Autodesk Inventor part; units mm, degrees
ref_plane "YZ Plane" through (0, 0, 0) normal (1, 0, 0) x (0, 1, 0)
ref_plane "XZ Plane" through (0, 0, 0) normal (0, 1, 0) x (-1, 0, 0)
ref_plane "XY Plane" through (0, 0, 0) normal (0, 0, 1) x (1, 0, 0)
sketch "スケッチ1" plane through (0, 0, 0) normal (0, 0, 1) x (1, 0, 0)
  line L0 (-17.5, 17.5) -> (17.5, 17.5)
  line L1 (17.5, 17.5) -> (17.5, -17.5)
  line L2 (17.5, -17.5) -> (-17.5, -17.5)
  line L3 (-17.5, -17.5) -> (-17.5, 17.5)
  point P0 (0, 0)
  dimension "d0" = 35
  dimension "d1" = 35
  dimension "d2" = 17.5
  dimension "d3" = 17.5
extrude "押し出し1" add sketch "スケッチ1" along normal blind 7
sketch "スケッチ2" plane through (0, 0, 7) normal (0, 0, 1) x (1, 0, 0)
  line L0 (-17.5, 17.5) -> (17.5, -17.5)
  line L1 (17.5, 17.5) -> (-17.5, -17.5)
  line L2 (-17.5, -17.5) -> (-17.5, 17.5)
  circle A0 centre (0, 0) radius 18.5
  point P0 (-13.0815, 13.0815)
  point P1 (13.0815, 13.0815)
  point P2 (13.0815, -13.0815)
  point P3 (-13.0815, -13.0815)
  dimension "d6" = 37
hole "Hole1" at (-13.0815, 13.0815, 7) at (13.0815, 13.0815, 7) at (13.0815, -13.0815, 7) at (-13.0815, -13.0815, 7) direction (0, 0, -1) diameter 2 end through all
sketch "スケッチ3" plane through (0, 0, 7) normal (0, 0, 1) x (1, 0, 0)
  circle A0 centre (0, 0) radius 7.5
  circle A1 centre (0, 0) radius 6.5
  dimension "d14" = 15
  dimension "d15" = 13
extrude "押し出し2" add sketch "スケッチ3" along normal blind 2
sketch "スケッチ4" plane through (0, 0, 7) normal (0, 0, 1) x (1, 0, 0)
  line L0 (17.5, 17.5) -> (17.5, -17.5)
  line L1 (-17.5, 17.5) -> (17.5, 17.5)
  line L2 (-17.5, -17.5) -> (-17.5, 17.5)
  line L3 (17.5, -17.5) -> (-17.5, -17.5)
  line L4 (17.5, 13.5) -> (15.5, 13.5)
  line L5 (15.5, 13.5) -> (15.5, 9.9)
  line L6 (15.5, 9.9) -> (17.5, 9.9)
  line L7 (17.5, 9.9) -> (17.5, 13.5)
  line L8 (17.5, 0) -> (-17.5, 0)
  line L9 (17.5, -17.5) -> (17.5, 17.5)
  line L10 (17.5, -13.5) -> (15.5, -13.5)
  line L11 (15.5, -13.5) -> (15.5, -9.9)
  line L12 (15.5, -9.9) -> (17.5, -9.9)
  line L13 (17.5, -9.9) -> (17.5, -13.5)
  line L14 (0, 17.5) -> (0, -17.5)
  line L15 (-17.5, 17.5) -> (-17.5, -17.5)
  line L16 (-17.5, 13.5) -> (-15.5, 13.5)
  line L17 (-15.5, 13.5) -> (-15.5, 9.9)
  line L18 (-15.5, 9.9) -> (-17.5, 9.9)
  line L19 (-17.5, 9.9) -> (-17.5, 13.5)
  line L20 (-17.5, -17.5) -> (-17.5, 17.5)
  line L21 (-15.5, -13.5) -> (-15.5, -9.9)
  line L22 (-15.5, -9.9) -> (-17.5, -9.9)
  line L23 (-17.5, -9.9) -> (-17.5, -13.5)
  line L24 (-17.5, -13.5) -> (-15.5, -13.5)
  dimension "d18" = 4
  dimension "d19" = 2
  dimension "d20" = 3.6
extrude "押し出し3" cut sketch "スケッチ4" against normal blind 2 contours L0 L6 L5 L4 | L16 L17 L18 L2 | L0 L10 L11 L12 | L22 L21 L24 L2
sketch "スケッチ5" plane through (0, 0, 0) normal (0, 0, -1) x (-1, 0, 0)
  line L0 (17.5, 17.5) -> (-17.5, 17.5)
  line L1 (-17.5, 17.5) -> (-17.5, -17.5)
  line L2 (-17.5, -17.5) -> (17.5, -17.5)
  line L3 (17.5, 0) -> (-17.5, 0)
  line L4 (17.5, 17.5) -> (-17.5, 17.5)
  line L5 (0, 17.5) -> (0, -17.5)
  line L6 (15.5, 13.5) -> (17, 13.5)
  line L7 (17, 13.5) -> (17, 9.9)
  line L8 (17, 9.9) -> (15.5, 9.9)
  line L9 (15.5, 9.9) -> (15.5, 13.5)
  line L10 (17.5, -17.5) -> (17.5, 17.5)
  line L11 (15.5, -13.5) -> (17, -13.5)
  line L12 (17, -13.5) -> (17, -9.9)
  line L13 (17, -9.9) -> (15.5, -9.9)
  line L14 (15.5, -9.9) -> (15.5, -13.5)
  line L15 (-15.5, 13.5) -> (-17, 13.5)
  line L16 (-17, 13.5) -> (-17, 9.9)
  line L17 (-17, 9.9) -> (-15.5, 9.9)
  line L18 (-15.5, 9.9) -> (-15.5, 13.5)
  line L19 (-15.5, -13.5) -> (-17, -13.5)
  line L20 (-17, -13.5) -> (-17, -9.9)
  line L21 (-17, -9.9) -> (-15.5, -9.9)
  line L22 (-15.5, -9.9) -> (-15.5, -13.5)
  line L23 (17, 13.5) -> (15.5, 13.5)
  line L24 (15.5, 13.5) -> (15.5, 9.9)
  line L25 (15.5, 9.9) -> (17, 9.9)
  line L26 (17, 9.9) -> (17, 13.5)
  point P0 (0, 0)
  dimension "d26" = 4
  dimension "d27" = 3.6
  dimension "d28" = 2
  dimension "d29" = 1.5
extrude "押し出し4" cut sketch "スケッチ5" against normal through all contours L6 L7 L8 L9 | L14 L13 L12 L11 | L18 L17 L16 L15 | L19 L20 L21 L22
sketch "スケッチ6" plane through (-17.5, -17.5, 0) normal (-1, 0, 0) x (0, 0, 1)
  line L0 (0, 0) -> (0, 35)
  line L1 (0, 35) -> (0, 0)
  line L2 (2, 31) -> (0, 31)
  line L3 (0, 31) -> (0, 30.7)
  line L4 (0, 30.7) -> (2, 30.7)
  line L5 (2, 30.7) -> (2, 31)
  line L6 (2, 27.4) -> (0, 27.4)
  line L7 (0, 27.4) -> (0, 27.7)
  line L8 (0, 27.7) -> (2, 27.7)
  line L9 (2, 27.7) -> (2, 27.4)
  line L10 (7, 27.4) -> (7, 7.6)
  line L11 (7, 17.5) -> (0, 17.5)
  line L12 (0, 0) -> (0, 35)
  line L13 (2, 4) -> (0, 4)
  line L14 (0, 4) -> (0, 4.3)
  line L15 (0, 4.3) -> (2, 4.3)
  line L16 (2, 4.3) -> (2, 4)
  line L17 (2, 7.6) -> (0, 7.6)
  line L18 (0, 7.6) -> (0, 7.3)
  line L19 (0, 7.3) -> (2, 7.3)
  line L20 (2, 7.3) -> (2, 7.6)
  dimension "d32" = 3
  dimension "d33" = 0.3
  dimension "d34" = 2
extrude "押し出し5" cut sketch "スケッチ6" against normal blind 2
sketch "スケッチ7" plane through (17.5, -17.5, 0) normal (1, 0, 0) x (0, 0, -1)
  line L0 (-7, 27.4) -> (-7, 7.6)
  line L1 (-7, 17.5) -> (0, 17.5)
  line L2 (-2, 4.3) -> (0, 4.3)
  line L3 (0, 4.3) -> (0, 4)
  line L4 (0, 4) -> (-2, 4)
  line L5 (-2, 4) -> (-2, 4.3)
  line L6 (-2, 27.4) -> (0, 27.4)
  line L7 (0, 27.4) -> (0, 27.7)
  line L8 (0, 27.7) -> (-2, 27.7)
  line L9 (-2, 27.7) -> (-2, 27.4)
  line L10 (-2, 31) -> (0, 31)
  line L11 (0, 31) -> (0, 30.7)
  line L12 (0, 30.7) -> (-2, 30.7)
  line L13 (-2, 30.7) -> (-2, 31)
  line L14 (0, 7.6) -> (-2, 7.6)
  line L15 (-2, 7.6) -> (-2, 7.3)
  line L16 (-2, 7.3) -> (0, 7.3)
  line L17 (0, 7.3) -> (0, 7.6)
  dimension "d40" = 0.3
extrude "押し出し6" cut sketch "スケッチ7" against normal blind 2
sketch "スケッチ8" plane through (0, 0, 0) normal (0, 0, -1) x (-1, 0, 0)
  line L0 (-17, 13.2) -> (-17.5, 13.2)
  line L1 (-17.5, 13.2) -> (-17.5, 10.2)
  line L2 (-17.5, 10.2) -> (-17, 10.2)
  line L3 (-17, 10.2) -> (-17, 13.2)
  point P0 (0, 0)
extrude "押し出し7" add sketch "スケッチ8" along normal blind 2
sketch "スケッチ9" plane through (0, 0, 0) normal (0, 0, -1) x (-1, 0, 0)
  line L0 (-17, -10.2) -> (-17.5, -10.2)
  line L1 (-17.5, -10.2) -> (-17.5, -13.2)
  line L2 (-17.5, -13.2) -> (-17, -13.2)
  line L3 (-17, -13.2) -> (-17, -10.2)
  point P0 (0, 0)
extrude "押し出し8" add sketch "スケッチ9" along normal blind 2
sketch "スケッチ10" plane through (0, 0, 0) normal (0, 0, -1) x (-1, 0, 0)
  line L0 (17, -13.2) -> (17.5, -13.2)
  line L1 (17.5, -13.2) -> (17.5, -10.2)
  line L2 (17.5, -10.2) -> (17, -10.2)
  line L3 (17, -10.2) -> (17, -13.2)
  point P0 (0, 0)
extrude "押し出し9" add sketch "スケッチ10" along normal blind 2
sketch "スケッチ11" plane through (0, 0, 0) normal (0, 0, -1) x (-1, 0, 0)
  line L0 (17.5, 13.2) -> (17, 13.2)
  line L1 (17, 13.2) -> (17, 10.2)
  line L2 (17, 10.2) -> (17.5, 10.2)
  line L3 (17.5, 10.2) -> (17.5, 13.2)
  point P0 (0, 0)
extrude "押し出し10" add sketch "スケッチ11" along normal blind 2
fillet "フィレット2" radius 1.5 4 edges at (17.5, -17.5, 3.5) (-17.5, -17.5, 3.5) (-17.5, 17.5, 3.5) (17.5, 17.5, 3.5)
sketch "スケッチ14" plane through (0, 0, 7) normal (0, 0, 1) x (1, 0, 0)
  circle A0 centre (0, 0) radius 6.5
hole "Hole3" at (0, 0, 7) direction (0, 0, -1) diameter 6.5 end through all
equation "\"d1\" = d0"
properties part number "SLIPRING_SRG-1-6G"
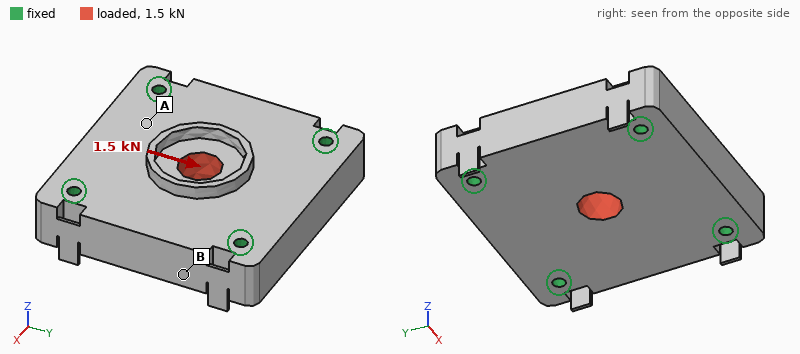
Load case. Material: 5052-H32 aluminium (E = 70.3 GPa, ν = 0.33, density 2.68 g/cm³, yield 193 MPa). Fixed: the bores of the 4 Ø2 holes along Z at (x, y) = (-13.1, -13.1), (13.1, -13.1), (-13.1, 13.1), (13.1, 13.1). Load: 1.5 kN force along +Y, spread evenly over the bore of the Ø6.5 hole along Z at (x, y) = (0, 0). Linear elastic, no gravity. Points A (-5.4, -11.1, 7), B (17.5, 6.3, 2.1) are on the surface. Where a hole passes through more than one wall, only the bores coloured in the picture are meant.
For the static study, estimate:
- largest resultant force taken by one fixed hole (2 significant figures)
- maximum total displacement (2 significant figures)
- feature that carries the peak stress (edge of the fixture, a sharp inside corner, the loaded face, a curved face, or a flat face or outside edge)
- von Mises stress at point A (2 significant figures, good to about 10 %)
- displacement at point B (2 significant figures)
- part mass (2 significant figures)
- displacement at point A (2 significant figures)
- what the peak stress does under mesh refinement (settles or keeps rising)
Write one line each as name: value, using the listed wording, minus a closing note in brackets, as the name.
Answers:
largest resultant force taken by one fixed hole: 410 N
maximum total displacement: 2.3 µm
feature that carries the peak stress: edge of the fixture
von Mises stress at point A: 5.1 MPa
displacement at point B: 0.39 µm
part mass: 22 g
displacement at point A: 1.3 µm
what the peak stress does under mesh refinement: keeps rising
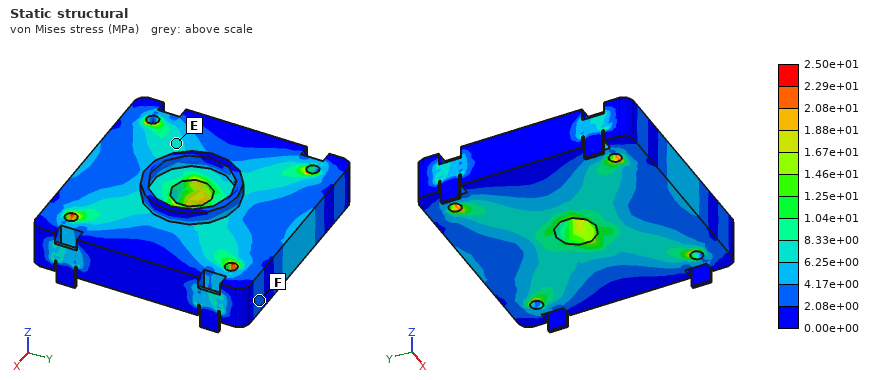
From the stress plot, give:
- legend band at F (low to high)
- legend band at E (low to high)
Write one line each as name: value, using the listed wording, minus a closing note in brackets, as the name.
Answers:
legend band at F: 2.08e+00 to 4.17e+00 MPa
legend band at E: 6.25e+00 to 8.33e+00 MPa
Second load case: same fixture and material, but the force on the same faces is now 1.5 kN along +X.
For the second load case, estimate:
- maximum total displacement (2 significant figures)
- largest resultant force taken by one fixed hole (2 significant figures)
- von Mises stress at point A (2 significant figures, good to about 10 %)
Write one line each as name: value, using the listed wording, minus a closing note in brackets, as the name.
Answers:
maximum total displacement: 2.4 µm
largest resultant force taken by one fixed hole: 410 N
von Mises stress at point A: 5.1 MPa
